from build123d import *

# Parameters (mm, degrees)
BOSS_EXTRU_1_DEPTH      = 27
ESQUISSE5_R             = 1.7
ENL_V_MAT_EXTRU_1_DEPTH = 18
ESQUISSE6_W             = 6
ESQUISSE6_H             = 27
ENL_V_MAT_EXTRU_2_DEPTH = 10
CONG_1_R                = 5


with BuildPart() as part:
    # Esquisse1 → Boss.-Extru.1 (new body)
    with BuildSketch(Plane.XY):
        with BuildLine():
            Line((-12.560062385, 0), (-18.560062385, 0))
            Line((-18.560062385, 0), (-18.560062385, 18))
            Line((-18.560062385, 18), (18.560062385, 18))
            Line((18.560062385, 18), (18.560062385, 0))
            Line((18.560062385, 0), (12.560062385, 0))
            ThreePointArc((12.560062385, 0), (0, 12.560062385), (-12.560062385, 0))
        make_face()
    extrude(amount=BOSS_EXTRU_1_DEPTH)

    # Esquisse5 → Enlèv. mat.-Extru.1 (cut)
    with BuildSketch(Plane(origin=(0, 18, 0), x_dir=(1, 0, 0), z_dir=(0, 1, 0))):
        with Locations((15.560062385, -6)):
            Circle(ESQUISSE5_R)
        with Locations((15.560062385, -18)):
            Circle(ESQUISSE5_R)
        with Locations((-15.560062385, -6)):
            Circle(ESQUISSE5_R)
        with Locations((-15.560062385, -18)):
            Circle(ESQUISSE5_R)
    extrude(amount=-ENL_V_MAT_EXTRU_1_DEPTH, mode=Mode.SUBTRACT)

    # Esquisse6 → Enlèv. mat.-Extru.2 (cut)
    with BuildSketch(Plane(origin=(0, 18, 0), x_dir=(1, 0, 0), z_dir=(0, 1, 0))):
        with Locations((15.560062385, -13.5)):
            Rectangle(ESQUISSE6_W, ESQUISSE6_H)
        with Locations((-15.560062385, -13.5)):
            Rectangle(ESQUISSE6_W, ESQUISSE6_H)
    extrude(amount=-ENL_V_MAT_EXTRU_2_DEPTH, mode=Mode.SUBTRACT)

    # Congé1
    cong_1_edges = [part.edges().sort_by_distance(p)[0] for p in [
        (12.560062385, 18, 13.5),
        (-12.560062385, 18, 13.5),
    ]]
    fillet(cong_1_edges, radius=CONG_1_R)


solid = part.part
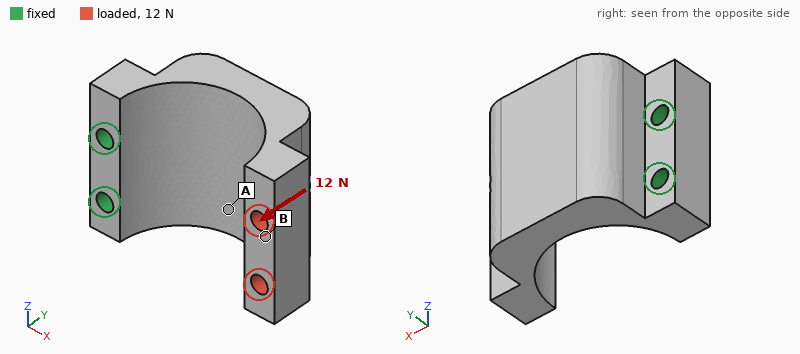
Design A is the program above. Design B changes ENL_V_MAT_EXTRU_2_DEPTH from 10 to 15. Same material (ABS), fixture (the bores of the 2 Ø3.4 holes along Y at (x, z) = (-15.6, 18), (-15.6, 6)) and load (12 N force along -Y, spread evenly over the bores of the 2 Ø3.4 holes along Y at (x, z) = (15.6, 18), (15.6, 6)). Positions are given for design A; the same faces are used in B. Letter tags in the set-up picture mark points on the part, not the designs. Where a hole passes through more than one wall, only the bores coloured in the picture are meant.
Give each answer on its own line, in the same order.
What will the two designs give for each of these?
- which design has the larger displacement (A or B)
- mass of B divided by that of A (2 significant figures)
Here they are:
B
0.81
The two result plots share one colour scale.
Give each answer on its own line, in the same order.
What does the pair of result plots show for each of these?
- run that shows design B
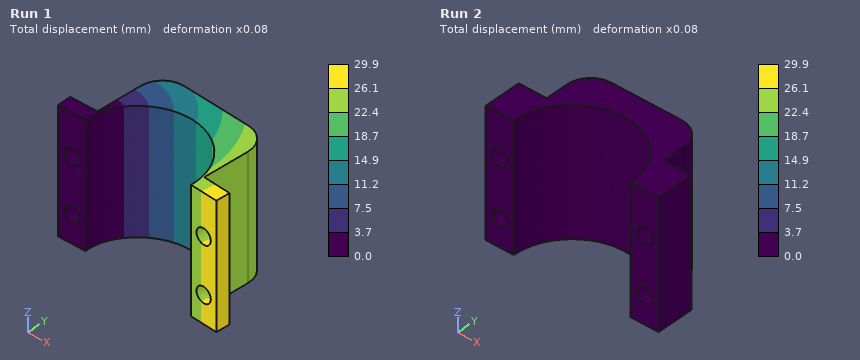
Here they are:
Run 1
